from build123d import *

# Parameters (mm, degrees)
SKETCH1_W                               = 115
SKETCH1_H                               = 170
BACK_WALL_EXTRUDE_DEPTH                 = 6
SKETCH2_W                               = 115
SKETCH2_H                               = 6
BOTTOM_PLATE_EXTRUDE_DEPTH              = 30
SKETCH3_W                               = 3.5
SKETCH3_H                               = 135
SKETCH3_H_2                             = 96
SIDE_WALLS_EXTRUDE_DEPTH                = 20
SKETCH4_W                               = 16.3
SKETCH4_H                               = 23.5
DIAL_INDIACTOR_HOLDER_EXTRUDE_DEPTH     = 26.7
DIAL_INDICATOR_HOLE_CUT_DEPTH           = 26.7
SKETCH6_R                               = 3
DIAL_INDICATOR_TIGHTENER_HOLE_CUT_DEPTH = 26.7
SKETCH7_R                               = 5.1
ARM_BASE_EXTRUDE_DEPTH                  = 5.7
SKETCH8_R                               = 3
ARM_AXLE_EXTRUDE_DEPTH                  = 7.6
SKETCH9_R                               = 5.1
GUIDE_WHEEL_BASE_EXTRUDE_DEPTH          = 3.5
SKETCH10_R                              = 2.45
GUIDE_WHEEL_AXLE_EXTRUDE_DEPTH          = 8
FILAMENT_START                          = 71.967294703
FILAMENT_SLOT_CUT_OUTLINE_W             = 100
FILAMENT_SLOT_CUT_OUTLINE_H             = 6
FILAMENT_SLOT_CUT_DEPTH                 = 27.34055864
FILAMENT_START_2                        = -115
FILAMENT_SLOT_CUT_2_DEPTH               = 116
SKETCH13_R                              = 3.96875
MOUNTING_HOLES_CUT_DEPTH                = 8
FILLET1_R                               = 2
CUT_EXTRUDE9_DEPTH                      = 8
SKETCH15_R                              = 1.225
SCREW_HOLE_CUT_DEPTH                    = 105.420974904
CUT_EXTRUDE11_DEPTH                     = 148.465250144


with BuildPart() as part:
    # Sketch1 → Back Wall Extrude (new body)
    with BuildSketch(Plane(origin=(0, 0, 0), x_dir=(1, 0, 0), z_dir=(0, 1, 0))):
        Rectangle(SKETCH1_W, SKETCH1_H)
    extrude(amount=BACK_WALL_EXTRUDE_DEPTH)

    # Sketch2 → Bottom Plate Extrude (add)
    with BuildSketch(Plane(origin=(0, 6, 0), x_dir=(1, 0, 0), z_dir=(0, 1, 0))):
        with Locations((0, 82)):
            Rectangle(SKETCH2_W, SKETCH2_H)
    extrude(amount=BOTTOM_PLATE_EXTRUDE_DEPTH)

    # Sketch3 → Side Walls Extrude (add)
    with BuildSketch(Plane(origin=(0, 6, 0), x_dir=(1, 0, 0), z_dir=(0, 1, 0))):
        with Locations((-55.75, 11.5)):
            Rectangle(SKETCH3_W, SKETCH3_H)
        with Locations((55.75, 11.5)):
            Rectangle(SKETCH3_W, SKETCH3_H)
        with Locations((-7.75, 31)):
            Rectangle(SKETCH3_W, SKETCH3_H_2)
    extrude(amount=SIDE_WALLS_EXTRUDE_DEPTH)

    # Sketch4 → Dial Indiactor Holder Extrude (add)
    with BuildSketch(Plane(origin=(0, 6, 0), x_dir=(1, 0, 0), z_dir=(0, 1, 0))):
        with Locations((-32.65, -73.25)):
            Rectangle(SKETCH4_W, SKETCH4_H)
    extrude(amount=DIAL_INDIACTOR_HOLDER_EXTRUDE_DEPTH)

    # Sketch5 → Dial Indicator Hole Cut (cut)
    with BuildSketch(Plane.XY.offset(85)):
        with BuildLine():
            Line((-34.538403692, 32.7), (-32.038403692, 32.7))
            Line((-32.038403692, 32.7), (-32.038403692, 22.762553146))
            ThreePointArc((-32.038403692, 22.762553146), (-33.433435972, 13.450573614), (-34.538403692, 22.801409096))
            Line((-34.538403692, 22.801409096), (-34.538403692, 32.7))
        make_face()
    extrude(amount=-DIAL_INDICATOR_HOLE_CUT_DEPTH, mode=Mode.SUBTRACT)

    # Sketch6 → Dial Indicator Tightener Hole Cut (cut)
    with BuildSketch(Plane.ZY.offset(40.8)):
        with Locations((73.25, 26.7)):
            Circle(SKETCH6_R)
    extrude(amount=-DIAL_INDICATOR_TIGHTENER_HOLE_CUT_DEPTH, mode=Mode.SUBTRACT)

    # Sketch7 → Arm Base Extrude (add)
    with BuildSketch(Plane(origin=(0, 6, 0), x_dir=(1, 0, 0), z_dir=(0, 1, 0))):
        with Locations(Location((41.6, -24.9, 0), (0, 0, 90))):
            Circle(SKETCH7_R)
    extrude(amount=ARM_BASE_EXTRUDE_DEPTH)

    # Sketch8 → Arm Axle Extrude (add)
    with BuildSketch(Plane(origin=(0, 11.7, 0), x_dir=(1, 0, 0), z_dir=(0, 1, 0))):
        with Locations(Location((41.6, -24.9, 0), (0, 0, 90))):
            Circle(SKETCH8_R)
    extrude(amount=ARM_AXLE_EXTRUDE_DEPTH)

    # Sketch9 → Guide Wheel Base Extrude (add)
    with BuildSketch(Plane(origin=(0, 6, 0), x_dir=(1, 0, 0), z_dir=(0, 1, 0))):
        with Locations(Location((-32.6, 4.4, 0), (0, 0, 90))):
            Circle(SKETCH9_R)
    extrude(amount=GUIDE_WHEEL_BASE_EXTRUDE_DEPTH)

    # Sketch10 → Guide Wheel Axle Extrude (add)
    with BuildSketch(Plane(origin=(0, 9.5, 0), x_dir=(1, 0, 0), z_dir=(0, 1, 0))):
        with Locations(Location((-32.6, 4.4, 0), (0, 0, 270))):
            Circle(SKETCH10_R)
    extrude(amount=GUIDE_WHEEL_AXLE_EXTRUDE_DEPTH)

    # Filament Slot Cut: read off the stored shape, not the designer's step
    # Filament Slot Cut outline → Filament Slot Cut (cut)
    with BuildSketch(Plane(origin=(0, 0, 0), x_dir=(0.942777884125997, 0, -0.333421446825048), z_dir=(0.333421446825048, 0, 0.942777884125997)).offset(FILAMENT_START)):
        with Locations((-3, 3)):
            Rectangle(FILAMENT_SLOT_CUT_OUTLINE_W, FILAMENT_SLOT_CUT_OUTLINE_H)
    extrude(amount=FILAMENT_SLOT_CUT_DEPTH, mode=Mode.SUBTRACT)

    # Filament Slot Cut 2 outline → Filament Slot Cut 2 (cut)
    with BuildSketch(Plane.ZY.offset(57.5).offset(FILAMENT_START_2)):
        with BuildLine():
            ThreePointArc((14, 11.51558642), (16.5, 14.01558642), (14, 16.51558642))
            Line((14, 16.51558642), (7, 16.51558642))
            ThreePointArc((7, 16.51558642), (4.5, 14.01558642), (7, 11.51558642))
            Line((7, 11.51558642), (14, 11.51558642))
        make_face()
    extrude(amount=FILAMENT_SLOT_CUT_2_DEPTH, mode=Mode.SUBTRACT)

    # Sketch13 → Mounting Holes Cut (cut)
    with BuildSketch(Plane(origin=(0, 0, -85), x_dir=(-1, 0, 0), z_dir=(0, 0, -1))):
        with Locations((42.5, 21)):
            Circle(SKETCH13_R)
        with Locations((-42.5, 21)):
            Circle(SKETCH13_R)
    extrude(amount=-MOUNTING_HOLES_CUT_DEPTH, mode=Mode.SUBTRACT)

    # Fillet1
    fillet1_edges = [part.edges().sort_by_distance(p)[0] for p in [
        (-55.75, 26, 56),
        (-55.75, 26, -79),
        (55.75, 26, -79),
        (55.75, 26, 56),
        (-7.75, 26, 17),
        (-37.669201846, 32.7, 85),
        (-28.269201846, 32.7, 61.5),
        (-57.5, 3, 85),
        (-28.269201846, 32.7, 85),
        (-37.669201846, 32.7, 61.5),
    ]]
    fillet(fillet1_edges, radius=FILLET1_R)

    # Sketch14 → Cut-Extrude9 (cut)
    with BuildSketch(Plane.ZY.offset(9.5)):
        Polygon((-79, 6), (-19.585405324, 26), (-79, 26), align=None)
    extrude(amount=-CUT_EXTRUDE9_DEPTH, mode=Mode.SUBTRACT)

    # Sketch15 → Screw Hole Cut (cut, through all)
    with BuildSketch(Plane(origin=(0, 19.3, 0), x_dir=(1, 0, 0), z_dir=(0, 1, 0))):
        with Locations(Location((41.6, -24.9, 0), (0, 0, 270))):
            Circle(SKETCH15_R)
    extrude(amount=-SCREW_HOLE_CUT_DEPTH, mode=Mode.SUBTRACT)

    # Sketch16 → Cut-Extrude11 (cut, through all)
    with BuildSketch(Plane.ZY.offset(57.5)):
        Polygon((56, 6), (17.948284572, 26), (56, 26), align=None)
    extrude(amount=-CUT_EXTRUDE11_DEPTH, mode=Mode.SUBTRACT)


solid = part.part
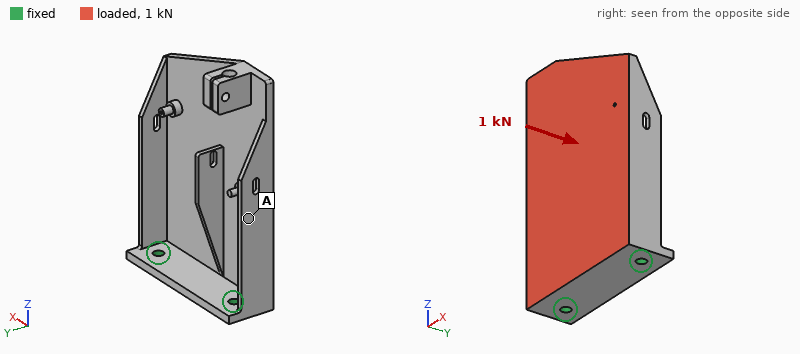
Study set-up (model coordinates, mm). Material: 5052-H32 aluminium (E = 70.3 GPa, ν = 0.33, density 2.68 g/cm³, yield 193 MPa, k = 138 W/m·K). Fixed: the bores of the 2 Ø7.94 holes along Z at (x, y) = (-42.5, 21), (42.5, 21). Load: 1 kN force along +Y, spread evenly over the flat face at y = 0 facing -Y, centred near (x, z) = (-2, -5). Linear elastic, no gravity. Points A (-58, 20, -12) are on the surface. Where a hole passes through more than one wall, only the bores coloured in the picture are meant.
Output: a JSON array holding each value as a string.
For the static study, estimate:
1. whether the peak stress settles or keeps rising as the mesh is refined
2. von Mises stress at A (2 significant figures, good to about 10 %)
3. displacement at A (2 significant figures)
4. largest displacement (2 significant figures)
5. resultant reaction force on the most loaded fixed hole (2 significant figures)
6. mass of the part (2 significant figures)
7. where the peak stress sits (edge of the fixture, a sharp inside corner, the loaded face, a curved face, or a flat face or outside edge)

["keeps rising", "14 MPa", "0.45 mm", "1.3 mm", "520 N", "430 g", "a sharp inside corner"]
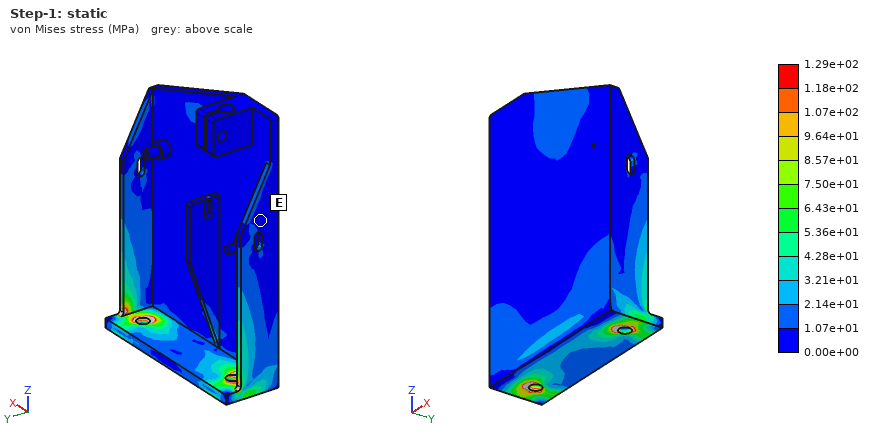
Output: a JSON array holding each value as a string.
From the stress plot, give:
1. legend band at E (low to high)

["0.00e+00 to 1.07e+01 MPa"]
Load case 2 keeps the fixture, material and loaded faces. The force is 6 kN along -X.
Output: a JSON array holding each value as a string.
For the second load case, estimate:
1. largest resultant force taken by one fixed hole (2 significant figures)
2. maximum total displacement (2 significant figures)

["6.0 kN", "0.79 mm"]
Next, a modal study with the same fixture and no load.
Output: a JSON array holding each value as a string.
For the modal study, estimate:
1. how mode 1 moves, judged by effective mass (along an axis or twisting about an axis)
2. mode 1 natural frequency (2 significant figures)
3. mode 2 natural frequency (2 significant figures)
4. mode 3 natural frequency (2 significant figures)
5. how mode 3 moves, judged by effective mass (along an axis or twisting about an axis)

["along Y", "290 Hz", "600 Hz", "1400 Hz", "along X"]
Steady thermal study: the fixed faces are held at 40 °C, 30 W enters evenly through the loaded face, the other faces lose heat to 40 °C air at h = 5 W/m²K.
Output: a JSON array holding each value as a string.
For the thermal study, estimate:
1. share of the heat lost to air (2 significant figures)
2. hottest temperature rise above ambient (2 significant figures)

["11 %", "24 K"]
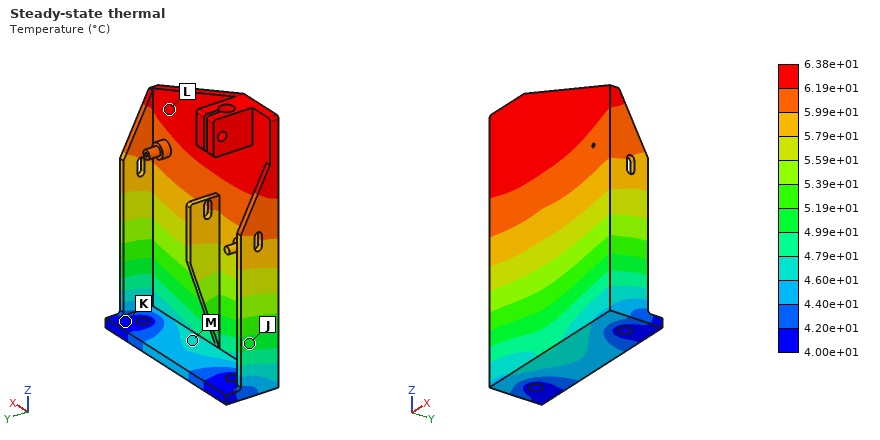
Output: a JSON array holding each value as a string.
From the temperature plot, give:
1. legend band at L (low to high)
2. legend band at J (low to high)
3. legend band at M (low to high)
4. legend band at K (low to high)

["6.19e+01 to 6.38e+01 °C", "4.99e+01 to 5.19e+01 °C", "4.60e+01 to 4.79e+01 °C", "4.00e+01 to 4.20e+01 °C"]
